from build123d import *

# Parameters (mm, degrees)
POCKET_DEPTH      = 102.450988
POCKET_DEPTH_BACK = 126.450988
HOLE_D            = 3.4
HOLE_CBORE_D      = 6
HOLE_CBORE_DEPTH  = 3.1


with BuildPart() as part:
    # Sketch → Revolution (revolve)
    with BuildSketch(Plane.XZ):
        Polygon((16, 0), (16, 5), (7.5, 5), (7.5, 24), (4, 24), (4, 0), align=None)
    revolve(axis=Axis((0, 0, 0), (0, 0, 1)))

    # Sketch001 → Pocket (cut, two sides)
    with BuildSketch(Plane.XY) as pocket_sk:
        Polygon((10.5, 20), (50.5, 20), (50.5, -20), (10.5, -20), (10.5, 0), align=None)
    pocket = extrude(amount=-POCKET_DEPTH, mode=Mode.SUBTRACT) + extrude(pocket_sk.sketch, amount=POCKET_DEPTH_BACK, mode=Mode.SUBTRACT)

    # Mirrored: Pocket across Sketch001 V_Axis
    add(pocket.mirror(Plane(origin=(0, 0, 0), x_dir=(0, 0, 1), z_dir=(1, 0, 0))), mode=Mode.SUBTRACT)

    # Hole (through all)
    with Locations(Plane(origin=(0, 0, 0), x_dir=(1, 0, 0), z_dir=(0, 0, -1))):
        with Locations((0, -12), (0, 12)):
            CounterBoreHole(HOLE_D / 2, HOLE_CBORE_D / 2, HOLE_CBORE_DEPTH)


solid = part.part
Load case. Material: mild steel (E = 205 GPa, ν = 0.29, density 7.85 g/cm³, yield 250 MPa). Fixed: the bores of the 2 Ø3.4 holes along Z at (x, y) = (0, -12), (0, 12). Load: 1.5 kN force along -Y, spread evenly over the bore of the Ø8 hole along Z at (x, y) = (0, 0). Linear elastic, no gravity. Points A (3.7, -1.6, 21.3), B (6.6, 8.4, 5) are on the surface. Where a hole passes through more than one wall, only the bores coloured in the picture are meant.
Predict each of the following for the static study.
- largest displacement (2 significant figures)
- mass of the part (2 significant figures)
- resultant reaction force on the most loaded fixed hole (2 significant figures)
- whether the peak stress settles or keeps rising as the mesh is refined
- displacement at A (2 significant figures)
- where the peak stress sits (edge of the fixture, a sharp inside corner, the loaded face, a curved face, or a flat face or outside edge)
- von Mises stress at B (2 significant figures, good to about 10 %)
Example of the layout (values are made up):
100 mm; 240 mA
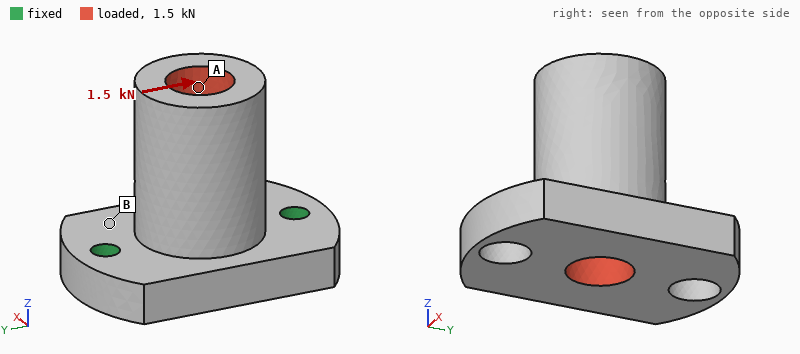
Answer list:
12 µm; 40 g; 940 N; keeps rising; 10.0 µm; edge of the fixture; 24 MPa
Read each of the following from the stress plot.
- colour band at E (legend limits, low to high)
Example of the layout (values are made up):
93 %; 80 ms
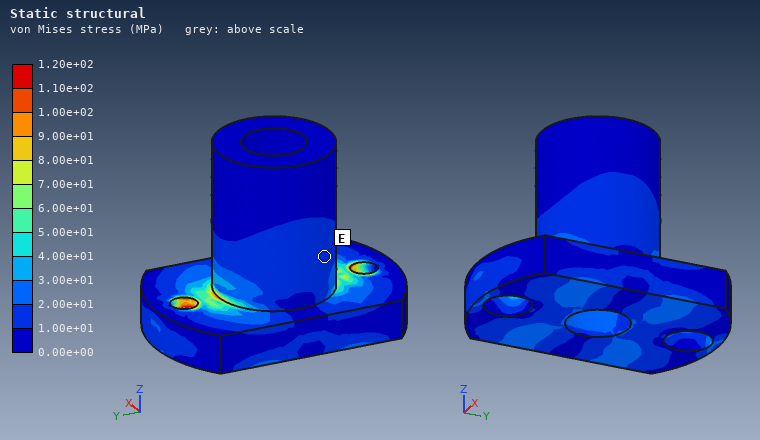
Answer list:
1.00e+01 to 2.00e+01 MPa
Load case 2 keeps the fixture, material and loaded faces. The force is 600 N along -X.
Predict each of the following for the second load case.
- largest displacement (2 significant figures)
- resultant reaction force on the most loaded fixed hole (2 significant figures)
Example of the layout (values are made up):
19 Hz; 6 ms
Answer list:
28 µm; 300 N
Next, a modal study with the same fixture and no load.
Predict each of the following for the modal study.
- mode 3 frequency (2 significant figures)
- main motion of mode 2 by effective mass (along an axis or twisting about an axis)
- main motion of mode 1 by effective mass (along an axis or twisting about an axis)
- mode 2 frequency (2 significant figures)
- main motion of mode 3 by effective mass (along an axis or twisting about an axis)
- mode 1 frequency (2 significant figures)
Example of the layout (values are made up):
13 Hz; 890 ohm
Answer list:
16 kHz; along Y; along X; 14 kHz; along Z; 5100 Hz
